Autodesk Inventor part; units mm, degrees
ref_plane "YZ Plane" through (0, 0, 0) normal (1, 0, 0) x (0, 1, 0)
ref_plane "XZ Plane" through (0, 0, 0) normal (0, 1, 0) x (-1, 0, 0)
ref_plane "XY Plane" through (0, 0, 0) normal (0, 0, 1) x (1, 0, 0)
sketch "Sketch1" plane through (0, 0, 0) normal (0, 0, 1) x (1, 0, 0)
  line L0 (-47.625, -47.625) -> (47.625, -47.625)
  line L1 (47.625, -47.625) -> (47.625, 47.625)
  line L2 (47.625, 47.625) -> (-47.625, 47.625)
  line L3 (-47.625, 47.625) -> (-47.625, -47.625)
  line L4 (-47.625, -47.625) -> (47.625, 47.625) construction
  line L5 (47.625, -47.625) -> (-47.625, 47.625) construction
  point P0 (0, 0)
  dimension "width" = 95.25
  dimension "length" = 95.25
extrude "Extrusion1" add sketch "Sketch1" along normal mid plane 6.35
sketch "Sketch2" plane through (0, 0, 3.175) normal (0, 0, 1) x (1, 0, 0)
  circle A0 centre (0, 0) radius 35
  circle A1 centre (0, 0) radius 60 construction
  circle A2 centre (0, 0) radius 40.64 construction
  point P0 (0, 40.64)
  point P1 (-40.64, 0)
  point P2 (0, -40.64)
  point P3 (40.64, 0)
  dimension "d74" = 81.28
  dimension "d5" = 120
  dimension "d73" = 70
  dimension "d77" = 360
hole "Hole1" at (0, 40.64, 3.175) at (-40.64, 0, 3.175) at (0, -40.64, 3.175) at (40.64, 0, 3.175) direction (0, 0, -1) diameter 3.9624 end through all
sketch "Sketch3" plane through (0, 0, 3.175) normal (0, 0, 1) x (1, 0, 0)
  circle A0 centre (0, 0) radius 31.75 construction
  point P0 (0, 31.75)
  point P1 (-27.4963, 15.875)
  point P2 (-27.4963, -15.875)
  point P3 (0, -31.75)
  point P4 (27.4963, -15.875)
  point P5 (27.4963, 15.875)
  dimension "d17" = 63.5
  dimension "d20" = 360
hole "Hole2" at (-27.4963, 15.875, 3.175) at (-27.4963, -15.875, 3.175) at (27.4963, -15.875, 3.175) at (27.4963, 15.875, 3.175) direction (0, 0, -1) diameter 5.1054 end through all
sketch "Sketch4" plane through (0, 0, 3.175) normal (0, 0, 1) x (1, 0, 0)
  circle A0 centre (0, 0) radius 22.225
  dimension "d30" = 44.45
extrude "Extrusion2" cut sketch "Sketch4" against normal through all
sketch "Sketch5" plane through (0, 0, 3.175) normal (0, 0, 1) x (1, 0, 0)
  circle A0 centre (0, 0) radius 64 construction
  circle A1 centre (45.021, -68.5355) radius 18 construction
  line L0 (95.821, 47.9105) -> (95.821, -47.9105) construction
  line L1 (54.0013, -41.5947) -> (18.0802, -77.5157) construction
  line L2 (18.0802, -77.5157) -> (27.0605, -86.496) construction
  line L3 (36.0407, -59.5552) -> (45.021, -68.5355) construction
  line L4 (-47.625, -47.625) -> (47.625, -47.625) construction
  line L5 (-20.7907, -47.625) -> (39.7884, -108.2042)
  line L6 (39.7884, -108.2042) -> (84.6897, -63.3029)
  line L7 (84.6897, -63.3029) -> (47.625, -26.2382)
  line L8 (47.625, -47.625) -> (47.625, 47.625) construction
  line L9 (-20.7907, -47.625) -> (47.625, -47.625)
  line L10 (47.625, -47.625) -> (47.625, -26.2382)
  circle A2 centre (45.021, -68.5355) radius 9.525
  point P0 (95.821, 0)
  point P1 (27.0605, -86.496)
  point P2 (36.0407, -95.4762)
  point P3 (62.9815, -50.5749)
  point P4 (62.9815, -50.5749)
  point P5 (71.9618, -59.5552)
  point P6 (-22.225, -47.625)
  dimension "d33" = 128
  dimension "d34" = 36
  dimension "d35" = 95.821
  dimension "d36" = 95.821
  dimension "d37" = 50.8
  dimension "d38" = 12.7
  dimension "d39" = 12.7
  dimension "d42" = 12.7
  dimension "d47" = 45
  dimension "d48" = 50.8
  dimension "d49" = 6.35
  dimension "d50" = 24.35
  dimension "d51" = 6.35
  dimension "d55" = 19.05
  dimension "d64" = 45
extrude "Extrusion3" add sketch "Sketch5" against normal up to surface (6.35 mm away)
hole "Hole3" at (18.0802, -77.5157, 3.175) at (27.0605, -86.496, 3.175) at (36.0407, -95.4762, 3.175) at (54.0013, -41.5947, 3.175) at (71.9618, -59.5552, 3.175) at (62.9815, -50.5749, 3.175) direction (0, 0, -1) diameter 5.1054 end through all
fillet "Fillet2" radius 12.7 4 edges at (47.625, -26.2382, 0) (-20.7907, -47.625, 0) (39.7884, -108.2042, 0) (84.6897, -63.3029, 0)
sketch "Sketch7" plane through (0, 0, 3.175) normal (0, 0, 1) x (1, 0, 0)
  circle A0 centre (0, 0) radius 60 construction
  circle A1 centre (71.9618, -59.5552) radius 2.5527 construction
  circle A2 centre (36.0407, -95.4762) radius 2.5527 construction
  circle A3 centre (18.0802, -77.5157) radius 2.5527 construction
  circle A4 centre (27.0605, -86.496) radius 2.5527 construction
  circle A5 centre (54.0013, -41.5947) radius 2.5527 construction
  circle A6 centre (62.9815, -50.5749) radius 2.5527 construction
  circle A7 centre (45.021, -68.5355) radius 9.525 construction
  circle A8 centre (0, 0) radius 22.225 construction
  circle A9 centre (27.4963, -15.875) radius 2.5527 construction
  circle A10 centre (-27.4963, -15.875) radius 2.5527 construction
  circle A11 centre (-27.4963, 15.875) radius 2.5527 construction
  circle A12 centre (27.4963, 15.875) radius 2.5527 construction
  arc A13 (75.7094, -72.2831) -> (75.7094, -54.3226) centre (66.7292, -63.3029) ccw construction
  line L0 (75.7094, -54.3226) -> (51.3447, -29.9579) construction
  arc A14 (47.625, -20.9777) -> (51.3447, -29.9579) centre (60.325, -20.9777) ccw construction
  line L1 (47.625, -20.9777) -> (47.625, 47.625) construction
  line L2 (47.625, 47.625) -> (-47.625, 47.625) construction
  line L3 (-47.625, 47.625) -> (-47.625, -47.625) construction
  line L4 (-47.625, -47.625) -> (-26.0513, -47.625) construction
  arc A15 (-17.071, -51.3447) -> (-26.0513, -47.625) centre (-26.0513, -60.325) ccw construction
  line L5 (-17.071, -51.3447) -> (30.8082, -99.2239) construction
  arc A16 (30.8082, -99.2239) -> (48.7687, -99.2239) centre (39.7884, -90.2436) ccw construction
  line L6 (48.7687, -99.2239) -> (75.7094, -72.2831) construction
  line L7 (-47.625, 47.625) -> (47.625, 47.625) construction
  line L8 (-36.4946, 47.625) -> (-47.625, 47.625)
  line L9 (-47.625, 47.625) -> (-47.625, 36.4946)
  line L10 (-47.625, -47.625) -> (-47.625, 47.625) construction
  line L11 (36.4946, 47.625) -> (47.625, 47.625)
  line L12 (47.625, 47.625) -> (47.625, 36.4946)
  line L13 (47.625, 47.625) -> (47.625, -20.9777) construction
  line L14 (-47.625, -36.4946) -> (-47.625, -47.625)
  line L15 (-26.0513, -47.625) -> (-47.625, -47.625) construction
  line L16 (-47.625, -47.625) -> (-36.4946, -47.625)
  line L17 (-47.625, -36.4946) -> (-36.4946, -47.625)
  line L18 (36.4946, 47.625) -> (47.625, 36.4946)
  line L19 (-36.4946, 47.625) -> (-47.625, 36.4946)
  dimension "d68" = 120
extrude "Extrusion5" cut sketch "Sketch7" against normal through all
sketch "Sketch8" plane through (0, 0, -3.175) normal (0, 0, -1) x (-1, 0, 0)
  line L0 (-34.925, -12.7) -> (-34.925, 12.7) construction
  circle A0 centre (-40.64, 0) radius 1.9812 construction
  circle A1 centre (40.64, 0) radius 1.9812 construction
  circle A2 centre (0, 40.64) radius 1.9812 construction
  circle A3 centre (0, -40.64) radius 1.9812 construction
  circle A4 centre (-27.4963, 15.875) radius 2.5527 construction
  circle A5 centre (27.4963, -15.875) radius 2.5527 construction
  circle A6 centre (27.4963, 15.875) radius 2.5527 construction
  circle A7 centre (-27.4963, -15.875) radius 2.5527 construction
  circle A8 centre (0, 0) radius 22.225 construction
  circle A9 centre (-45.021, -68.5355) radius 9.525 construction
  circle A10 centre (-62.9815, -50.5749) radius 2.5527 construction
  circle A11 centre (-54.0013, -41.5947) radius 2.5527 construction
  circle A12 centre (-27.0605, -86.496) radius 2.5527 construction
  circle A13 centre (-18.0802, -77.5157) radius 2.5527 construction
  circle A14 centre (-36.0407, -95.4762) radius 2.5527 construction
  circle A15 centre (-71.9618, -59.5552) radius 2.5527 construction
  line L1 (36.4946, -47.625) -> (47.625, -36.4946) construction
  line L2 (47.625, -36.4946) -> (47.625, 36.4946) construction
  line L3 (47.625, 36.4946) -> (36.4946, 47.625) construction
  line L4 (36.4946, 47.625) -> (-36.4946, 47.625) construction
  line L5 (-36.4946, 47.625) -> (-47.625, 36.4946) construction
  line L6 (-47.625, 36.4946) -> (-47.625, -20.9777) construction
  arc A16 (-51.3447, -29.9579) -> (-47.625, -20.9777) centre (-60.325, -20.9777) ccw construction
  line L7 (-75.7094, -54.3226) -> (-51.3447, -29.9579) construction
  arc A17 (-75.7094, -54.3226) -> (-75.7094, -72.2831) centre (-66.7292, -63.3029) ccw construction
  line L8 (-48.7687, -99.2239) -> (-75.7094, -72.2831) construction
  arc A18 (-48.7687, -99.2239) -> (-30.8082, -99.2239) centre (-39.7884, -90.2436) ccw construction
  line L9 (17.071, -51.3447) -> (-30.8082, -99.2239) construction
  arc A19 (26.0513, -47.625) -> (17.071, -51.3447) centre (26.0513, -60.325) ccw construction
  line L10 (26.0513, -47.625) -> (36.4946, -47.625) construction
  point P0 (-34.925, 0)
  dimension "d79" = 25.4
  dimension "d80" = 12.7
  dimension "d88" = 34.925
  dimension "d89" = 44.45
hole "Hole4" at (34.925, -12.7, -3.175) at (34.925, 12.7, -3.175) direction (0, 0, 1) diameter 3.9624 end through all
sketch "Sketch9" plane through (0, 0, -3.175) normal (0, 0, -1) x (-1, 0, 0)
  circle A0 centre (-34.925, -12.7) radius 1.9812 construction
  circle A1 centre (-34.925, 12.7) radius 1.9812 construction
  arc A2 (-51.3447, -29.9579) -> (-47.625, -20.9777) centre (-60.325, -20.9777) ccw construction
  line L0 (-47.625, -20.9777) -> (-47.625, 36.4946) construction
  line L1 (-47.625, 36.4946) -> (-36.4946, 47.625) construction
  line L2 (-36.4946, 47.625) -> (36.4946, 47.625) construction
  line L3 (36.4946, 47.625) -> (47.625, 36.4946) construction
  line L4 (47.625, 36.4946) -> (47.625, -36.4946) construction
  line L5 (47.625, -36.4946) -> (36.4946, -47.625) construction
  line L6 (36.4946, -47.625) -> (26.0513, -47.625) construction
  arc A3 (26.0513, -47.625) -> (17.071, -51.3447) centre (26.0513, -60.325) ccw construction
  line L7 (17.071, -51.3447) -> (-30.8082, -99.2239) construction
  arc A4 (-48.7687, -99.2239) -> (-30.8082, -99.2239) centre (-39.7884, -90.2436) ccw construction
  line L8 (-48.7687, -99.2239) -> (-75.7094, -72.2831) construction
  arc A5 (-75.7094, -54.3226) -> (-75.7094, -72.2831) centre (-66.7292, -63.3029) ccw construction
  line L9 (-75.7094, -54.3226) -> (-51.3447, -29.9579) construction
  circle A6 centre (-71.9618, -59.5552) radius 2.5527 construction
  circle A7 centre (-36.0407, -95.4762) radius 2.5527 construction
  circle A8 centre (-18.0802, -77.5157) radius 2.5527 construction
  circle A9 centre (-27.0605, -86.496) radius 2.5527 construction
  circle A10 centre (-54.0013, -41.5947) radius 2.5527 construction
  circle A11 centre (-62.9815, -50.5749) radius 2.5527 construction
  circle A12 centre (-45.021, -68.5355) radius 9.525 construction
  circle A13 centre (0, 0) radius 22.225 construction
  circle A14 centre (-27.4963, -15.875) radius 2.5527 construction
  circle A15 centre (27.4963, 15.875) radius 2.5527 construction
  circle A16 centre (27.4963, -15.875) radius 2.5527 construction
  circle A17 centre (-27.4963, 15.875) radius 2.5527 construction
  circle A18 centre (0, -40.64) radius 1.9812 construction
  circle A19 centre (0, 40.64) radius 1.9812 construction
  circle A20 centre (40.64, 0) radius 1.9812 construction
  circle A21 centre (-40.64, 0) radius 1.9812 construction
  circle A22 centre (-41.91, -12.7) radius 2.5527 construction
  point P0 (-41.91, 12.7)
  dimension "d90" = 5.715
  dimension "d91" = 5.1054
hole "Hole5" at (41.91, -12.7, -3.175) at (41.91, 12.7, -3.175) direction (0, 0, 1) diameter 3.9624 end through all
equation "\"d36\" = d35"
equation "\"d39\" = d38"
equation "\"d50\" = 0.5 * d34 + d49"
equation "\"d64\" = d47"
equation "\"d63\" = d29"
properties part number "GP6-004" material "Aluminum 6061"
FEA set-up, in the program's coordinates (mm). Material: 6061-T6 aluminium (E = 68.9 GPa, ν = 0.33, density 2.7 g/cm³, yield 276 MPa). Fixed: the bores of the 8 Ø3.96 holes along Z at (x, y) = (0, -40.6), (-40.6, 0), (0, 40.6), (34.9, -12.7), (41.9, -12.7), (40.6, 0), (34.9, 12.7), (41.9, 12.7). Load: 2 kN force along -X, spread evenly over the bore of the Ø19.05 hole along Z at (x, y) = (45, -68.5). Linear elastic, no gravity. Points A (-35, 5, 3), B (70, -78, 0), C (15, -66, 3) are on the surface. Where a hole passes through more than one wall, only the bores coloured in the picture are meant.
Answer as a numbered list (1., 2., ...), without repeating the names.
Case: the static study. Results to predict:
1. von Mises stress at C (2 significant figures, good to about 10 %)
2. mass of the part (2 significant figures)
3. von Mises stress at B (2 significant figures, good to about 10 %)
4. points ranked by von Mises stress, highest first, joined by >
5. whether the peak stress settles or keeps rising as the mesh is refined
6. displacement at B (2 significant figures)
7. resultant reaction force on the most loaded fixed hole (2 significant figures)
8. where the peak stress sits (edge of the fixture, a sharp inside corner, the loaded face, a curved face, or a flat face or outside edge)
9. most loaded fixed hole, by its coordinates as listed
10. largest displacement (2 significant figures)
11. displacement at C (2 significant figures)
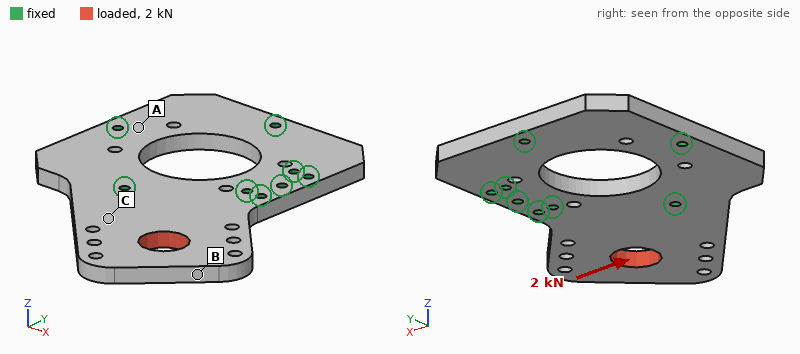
1. 9.6 MPa
2. 180 g
3. 6.3 MPa
4. C > B > A
5. keeps rising
6. 24 µm
7. 1.9 kN
8. edge of the fixture
9. (0, -40.6)
10. 24 µm
11. 10.0 µm
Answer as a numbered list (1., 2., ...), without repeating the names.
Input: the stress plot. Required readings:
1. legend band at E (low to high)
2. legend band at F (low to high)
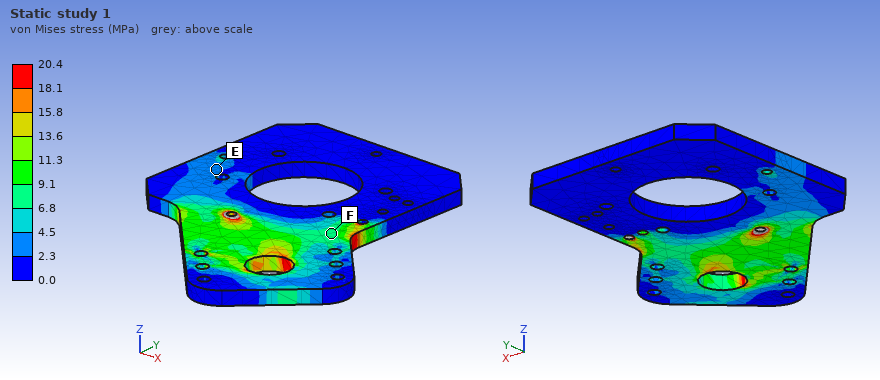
1. 2.3 to 4.5 MPa
2. 6.8 to 9.1 MPa
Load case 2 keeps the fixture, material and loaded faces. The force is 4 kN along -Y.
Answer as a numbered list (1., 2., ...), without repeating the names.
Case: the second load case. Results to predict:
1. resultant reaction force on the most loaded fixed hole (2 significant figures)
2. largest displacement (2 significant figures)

1. 1.9 kN
2. 42 µm
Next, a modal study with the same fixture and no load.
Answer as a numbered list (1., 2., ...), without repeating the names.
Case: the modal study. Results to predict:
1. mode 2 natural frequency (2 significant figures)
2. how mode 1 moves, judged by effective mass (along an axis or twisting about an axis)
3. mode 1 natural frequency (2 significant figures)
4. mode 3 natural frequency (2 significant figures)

1. 2700 Hz
2. along Z
3. 990 Hz
4. 4500 Hz
